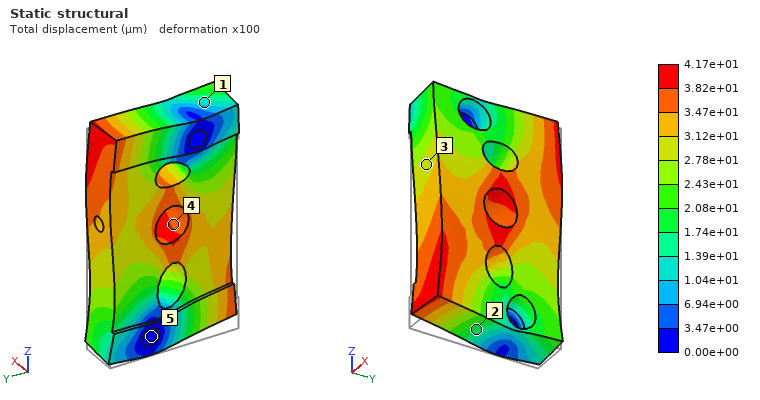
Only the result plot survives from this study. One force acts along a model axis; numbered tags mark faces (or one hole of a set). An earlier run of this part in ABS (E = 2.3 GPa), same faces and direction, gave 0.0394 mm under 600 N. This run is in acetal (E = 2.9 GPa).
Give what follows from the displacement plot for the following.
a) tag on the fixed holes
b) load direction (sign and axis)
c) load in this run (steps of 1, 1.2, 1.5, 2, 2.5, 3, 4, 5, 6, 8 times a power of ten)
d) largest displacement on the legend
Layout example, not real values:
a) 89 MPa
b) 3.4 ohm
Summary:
a) 5
b) +Z
c) 800 N
d) 4.17e+01 µm
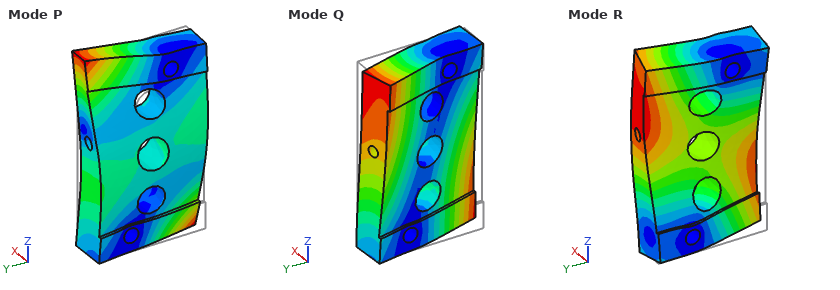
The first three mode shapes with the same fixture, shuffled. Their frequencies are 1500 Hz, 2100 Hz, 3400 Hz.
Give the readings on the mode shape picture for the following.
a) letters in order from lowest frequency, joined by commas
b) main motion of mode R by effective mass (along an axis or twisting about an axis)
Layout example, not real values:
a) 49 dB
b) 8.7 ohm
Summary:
a) Q, R, P
b) along X
